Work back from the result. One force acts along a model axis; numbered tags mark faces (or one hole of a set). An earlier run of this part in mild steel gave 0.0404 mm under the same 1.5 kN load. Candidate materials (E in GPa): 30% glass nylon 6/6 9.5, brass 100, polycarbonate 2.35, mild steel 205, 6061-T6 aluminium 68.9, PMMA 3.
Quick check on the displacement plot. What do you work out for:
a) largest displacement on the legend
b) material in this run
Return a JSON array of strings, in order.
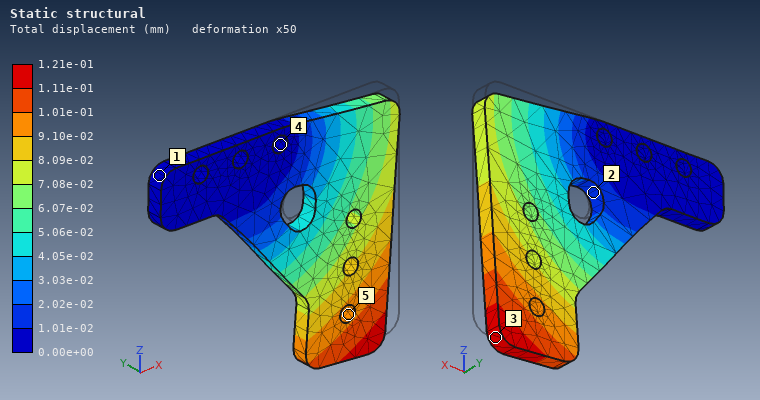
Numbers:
["1.21e-01 mm", "6061-T6 aluminium"]
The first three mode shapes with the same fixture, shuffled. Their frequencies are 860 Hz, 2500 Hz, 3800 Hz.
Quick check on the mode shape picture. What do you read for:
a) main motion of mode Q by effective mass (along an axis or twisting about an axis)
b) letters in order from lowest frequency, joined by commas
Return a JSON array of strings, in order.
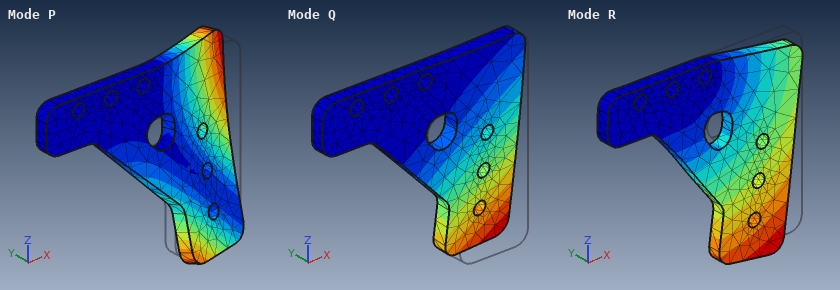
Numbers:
["along Y", "Q, P, R"]
